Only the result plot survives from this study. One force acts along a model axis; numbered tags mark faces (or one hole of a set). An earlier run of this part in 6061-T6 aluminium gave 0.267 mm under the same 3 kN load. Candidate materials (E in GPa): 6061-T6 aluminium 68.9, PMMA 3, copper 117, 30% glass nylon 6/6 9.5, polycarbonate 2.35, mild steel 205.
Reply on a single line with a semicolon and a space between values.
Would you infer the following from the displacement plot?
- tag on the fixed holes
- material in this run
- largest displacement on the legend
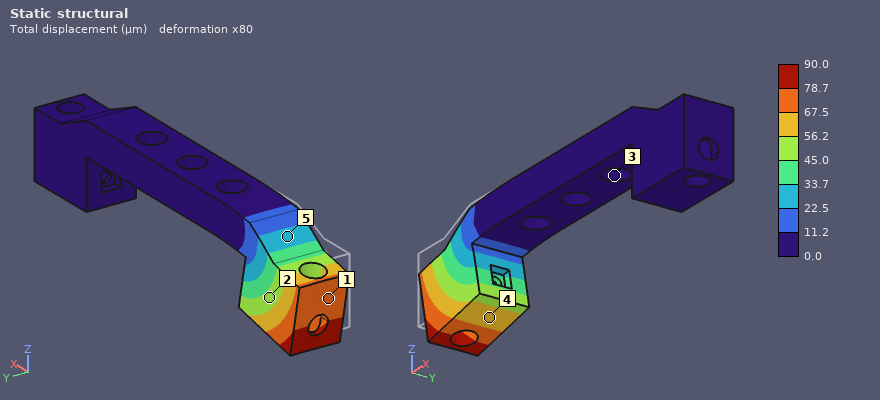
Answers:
3; mild steel; 90.0 µm
